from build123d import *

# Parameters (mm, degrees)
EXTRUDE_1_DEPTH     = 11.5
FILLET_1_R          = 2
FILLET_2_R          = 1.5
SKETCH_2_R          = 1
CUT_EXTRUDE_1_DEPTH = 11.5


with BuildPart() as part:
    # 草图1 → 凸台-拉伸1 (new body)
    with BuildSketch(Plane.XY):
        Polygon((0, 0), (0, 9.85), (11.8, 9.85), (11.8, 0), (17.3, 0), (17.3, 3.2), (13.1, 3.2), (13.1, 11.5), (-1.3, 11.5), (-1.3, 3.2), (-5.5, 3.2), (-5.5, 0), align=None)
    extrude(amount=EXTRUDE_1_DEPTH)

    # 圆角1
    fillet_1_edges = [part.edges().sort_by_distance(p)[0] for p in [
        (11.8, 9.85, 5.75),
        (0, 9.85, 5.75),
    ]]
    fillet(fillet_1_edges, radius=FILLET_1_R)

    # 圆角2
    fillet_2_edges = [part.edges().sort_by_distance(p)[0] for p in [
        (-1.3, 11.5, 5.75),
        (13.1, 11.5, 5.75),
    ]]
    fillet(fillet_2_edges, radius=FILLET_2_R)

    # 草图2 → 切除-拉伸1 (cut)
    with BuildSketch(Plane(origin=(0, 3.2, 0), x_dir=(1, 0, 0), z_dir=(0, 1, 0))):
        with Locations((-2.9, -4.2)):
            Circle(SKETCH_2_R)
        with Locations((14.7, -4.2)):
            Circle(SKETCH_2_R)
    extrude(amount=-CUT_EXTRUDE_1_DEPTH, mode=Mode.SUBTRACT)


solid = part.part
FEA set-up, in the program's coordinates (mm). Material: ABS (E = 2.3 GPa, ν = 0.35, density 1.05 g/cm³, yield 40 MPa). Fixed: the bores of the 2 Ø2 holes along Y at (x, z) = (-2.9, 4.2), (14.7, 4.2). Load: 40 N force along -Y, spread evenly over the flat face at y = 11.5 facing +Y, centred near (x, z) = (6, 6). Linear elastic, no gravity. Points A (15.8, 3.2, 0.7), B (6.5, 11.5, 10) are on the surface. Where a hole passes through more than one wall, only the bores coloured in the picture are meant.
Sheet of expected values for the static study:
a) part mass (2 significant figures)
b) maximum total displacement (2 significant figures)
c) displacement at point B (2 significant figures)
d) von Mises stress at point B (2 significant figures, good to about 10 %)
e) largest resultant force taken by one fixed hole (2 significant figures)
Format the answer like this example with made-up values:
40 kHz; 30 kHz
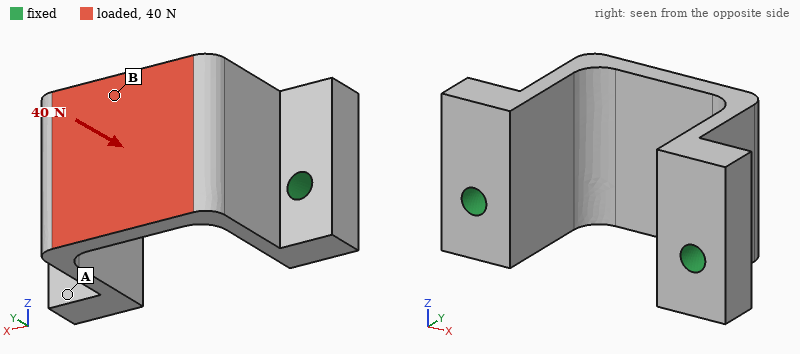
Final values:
0.91 g; 66 µm; 60 µm; 6.0 MPa; 21 N
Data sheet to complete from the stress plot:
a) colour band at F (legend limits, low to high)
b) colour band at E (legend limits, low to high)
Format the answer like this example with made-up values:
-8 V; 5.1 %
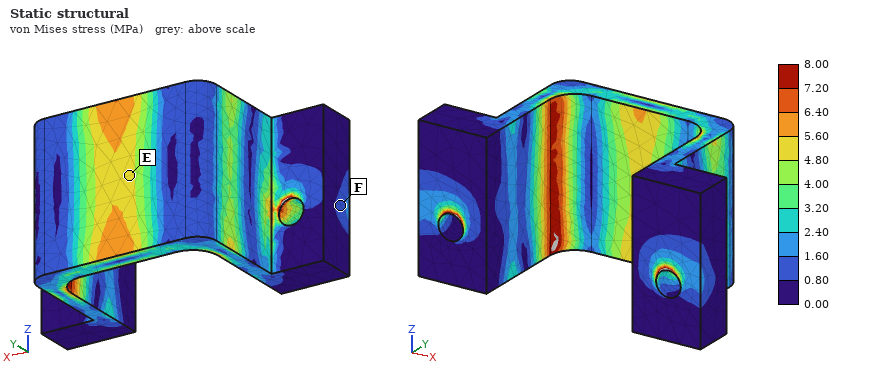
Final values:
0.80 to 1.60 MPa; 4.80 to 5.60 MPa
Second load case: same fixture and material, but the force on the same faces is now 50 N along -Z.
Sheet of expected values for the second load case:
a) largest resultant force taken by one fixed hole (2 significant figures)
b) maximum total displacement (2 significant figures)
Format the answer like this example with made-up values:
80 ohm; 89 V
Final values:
25 N; 0.17 mm
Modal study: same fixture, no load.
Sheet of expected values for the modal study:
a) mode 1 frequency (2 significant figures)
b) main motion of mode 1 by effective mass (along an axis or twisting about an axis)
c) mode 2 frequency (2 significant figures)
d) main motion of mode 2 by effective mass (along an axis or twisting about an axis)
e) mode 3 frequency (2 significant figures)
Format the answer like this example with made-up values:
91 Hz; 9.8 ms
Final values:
4000 Hz; along X; 5000 Hz; along Z; 6700 Hz
